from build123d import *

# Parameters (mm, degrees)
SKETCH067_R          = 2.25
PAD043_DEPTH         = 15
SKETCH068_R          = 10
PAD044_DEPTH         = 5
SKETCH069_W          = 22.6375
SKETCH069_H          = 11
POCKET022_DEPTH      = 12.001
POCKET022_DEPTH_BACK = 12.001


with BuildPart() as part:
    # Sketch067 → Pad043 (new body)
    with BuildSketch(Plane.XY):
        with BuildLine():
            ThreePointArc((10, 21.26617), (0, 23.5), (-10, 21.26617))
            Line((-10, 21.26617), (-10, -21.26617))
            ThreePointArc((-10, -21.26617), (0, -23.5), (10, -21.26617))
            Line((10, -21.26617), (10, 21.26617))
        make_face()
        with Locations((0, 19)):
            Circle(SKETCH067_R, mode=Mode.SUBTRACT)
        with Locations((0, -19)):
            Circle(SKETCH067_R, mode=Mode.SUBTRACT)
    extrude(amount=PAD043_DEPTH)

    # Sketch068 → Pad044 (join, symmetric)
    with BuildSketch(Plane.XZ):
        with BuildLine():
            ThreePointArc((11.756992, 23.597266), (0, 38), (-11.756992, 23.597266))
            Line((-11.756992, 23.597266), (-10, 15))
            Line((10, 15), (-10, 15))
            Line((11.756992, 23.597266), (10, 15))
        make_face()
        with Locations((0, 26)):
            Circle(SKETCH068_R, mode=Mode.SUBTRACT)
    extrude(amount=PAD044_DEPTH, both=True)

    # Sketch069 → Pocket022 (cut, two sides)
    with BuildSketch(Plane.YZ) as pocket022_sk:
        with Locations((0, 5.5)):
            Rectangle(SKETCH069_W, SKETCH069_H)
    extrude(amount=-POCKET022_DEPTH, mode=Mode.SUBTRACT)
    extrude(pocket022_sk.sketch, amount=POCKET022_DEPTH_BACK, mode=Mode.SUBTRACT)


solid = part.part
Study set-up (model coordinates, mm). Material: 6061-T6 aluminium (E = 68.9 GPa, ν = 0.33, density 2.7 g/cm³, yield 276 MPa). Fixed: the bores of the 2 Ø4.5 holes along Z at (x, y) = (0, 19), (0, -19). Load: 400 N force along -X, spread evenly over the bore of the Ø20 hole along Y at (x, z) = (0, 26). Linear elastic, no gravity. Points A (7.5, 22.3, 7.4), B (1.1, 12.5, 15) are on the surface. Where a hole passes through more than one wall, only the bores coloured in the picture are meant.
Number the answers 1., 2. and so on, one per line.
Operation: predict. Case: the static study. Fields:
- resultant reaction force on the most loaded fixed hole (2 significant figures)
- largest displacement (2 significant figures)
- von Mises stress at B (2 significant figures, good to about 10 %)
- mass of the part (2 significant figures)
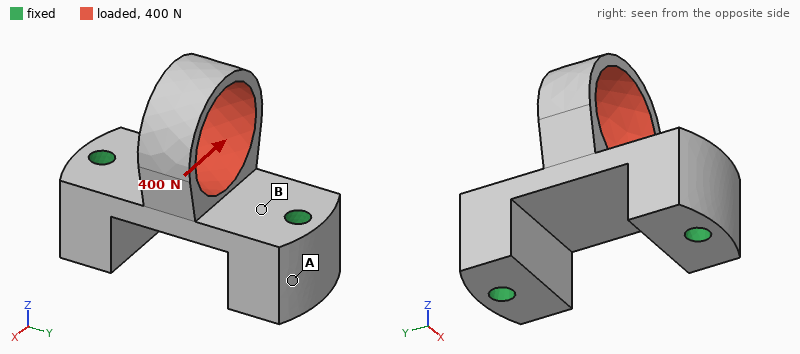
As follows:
1. 200 N
2. 0.10 mm
3. 15 MPa
4. 26 g
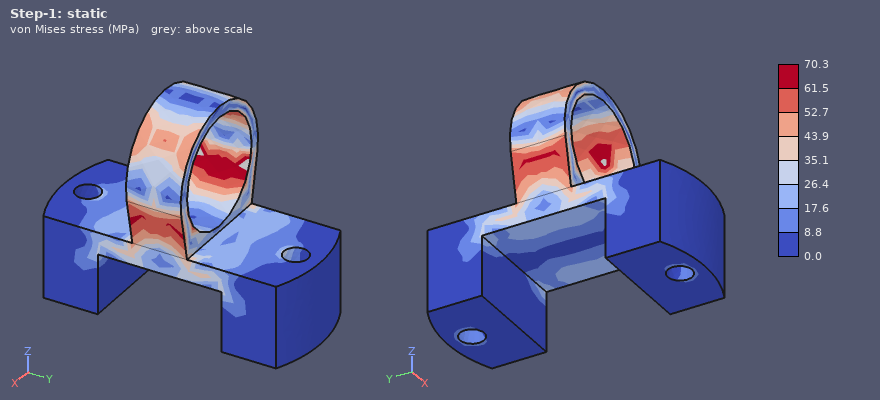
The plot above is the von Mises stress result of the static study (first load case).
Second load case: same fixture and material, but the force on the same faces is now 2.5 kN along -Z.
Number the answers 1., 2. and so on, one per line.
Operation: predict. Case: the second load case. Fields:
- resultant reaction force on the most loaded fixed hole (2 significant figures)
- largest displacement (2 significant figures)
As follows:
1. 1.6 kN
2. 0.11 mm
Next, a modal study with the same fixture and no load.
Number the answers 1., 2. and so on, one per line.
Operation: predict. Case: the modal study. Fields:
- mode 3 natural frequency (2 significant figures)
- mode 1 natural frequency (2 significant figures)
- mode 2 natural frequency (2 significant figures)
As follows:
1. 13 kHz
2. 5600 Hz
3. 8100 Hz
